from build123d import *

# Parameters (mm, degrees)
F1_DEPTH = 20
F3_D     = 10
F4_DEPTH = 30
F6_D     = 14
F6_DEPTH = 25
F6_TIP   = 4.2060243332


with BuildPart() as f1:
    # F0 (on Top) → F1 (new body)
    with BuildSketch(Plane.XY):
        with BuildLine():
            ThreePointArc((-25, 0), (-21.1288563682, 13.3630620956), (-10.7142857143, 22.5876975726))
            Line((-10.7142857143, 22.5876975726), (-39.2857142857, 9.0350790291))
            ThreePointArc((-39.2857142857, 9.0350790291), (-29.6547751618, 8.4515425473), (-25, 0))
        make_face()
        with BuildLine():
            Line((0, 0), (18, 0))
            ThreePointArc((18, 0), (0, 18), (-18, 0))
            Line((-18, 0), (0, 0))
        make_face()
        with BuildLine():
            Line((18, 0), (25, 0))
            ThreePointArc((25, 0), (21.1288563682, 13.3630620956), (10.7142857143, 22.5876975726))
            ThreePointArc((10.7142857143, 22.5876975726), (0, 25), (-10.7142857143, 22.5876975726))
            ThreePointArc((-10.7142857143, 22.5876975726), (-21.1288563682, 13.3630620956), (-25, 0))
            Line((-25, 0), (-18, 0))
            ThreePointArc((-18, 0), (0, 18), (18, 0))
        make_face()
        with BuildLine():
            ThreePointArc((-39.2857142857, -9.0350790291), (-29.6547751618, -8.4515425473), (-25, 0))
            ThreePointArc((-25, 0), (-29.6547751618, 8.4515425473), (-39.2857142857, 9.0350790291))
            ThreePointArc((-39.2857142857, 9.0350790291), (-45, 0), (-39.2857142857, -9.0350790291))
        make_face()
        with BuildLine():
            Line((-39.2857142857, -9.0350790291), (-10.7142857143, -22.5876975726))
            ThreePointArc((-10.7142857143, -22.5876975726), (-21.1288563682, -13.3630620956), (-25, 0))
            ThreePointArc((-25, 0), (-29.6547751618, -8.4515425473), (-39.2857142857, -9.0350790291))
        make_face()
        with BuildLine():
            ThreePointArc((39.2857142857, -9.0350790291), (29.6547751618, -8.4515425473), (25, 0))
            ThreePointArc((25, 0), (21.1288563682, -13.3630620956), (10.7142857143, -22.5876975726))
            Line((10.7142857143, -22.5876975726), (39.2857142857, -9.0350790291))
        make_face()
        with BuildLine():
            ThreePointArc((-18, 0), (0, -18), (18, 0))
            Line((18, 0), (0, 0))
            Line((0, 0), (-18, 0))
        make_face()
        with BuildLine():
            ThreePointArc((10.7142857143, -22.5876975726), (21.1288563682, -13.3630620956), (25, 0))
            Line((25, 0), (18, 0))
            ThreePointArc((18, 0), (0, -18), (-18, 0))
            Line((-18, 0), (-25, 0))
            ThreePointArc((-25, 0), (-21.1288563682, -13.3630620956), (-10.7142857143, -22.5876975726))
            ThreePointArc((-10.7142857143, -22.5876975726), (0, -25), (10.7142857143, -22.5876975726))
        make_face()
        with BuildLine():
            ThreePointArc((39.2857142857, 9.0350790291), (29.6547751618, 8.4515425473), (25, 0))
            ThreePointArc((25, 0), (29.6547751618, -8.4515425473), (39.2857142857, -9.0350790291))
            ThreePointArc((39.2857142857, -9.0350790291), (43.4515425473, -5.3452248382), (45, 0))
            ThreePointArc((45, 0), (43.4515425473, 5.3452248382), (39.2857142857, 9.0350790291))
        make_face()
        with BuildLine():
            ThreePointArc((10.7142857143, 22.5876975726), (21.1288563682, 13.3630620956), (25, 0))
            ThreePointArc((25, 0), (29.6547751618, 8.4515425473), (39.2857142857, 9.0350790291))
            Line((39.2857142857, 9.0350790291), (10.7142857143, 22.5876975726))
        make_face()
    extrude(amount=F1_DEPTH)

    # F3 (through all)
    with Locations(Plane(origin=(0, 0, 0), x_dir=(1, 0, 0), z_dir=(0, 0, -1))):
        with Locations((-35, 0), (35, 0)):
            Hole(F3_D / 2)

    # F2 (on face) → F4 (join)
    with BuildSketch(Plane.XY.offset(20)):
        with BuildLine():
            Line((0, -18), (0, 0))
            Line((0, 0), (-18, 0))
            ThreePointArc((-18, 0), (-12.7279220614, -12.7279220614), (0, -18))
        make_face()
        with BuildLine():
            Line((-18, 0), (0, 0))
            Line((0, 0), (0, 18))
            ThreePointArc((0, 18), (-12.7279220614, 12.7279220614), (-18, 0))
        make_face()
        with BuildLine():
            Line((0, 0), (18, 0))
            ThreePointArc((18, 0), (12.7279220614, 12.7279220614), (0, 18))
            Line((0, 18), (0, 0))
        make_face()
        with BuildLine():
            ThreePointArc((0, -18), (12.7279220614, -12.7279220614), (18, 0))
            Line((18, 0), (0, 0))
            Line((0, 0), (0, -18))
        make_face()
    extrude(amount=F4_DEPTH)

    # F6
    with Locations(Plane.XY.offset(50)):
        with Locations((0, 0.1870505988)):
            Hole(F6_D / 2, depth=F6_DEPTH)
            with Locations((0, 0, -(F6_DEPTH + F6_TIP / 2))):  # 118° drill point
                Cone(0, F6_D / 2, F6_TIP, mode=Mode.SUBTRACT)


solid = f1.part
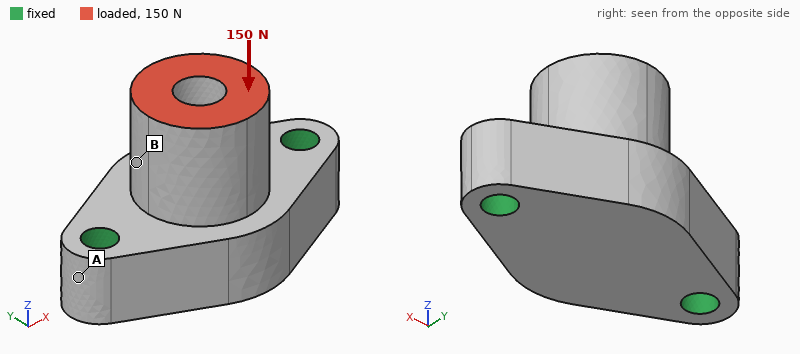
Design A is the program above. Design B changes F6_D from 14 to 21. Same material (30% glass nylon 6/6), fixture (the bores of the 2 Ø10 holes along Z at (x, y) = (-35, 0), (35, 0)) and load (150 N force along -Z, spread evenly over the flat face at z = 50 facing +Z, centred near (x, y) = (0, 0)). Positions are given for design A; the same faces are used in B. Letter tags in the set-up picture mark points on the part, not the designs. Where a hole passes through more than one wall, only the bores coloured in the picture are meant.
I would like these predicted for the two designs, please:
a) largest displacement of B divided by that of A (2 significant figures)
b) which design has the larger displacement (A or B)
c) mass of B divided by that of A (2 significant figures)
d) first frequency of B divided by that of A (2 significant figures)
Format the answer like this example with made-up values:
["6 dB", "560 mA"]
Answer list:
["1.1", "B", "0.94", "1.1"]
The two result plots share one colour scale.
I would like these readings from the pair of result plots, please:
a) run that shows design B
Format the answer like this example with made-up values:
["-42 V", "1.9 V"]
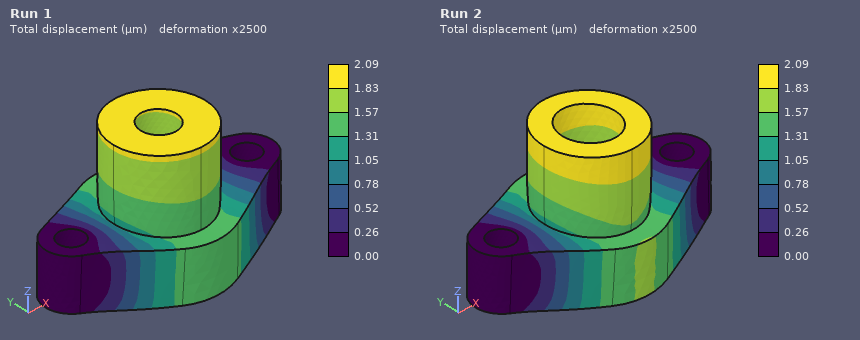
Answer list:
["Run 2"]
